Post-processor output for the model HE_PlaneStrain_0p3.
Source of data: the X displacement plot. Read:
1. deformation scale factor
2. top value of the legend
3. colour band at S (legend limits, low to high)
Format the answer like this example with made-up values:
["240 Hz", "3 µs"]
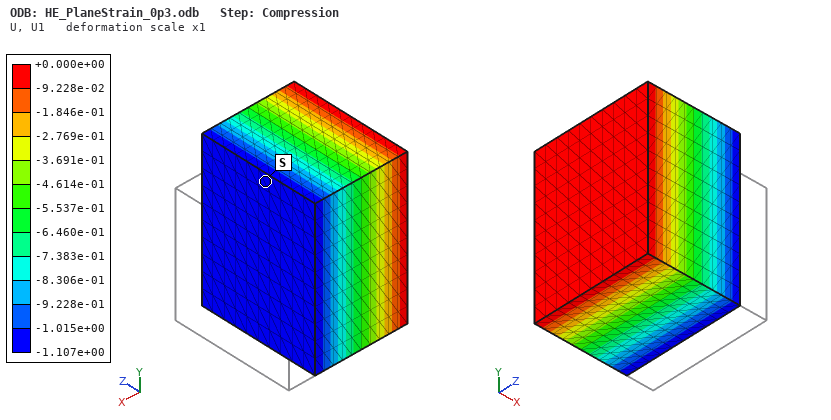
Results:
["1", "+0.000e+00", "-1.107e+00 to -1.015e+00"]
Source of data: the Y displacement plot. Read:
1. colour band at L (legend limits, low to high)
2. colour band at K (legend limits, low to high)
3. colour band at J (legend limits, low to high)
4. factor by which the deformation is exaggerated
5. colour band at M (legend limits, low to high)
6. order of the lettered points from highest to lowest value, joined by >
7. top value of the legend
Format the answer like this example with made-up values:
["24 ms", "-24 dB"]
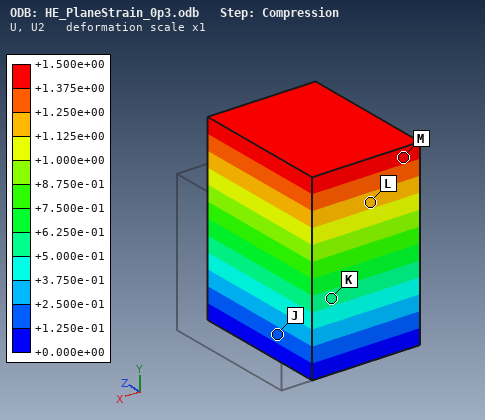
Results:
["+1.125e+00 to +1.250e+00", "+5.000e-01 to +6.250e-01", "+1.250e-01 to +2.500e-01", "1", "+1.375e+00 to +1.500e+00", "M > L > K > J", "+1.500e+00"]
